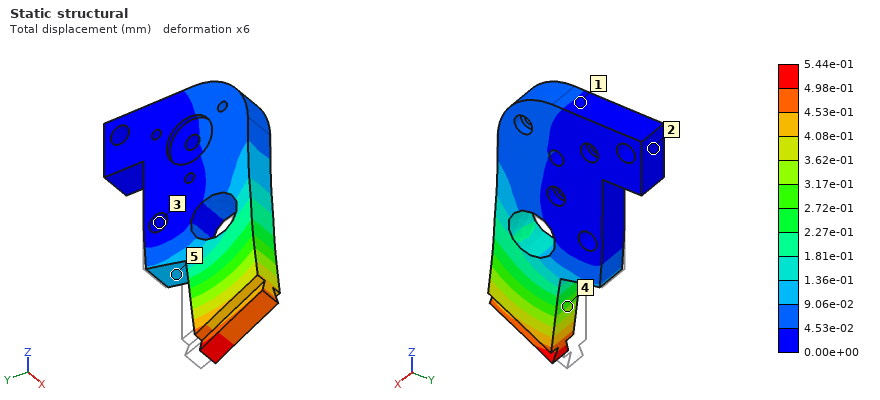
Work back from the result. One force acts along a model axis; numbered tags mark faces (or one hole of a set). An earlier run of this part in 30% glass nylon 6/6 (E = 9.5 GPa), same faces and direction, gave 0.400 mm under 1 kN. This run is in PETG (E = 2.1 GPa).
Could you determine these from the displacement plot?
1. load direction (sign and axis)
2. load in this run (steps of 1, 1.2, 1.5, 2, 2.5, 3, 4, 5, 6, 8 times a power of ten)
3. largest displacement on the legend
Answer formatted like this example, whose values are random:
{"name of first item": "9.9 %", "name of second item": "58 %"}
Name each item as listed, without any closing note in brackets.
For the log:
{"load direction": "-Y", "load in this run": "300 N", "largest displacement on the legend": "5.44e-01 mm"}
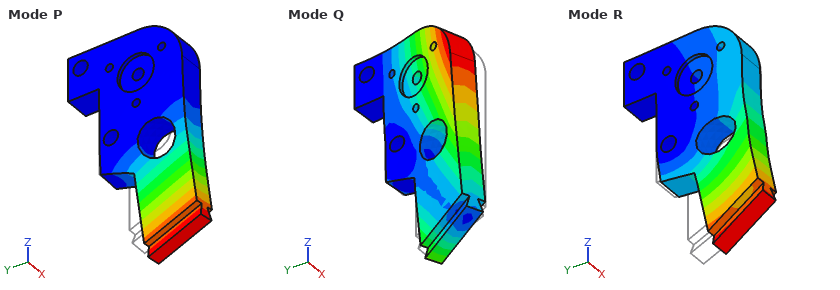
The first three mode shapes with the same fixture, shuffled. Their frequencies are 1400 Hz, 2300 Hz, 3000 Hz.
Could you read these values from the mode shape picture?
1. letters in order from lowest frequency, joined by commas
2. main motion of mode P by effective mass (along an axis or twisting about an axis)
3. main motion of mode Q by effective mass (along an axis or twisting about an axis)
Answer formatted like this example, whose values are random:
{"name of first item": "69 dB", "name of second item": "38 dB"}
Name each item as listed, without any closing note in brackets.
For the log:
{"letters in order from lowest frequency, joined by commas": "P, Q, R", "main motion of mode P by effective mass": "along X", "main motion of mode Q by effective mass": "along X"}
